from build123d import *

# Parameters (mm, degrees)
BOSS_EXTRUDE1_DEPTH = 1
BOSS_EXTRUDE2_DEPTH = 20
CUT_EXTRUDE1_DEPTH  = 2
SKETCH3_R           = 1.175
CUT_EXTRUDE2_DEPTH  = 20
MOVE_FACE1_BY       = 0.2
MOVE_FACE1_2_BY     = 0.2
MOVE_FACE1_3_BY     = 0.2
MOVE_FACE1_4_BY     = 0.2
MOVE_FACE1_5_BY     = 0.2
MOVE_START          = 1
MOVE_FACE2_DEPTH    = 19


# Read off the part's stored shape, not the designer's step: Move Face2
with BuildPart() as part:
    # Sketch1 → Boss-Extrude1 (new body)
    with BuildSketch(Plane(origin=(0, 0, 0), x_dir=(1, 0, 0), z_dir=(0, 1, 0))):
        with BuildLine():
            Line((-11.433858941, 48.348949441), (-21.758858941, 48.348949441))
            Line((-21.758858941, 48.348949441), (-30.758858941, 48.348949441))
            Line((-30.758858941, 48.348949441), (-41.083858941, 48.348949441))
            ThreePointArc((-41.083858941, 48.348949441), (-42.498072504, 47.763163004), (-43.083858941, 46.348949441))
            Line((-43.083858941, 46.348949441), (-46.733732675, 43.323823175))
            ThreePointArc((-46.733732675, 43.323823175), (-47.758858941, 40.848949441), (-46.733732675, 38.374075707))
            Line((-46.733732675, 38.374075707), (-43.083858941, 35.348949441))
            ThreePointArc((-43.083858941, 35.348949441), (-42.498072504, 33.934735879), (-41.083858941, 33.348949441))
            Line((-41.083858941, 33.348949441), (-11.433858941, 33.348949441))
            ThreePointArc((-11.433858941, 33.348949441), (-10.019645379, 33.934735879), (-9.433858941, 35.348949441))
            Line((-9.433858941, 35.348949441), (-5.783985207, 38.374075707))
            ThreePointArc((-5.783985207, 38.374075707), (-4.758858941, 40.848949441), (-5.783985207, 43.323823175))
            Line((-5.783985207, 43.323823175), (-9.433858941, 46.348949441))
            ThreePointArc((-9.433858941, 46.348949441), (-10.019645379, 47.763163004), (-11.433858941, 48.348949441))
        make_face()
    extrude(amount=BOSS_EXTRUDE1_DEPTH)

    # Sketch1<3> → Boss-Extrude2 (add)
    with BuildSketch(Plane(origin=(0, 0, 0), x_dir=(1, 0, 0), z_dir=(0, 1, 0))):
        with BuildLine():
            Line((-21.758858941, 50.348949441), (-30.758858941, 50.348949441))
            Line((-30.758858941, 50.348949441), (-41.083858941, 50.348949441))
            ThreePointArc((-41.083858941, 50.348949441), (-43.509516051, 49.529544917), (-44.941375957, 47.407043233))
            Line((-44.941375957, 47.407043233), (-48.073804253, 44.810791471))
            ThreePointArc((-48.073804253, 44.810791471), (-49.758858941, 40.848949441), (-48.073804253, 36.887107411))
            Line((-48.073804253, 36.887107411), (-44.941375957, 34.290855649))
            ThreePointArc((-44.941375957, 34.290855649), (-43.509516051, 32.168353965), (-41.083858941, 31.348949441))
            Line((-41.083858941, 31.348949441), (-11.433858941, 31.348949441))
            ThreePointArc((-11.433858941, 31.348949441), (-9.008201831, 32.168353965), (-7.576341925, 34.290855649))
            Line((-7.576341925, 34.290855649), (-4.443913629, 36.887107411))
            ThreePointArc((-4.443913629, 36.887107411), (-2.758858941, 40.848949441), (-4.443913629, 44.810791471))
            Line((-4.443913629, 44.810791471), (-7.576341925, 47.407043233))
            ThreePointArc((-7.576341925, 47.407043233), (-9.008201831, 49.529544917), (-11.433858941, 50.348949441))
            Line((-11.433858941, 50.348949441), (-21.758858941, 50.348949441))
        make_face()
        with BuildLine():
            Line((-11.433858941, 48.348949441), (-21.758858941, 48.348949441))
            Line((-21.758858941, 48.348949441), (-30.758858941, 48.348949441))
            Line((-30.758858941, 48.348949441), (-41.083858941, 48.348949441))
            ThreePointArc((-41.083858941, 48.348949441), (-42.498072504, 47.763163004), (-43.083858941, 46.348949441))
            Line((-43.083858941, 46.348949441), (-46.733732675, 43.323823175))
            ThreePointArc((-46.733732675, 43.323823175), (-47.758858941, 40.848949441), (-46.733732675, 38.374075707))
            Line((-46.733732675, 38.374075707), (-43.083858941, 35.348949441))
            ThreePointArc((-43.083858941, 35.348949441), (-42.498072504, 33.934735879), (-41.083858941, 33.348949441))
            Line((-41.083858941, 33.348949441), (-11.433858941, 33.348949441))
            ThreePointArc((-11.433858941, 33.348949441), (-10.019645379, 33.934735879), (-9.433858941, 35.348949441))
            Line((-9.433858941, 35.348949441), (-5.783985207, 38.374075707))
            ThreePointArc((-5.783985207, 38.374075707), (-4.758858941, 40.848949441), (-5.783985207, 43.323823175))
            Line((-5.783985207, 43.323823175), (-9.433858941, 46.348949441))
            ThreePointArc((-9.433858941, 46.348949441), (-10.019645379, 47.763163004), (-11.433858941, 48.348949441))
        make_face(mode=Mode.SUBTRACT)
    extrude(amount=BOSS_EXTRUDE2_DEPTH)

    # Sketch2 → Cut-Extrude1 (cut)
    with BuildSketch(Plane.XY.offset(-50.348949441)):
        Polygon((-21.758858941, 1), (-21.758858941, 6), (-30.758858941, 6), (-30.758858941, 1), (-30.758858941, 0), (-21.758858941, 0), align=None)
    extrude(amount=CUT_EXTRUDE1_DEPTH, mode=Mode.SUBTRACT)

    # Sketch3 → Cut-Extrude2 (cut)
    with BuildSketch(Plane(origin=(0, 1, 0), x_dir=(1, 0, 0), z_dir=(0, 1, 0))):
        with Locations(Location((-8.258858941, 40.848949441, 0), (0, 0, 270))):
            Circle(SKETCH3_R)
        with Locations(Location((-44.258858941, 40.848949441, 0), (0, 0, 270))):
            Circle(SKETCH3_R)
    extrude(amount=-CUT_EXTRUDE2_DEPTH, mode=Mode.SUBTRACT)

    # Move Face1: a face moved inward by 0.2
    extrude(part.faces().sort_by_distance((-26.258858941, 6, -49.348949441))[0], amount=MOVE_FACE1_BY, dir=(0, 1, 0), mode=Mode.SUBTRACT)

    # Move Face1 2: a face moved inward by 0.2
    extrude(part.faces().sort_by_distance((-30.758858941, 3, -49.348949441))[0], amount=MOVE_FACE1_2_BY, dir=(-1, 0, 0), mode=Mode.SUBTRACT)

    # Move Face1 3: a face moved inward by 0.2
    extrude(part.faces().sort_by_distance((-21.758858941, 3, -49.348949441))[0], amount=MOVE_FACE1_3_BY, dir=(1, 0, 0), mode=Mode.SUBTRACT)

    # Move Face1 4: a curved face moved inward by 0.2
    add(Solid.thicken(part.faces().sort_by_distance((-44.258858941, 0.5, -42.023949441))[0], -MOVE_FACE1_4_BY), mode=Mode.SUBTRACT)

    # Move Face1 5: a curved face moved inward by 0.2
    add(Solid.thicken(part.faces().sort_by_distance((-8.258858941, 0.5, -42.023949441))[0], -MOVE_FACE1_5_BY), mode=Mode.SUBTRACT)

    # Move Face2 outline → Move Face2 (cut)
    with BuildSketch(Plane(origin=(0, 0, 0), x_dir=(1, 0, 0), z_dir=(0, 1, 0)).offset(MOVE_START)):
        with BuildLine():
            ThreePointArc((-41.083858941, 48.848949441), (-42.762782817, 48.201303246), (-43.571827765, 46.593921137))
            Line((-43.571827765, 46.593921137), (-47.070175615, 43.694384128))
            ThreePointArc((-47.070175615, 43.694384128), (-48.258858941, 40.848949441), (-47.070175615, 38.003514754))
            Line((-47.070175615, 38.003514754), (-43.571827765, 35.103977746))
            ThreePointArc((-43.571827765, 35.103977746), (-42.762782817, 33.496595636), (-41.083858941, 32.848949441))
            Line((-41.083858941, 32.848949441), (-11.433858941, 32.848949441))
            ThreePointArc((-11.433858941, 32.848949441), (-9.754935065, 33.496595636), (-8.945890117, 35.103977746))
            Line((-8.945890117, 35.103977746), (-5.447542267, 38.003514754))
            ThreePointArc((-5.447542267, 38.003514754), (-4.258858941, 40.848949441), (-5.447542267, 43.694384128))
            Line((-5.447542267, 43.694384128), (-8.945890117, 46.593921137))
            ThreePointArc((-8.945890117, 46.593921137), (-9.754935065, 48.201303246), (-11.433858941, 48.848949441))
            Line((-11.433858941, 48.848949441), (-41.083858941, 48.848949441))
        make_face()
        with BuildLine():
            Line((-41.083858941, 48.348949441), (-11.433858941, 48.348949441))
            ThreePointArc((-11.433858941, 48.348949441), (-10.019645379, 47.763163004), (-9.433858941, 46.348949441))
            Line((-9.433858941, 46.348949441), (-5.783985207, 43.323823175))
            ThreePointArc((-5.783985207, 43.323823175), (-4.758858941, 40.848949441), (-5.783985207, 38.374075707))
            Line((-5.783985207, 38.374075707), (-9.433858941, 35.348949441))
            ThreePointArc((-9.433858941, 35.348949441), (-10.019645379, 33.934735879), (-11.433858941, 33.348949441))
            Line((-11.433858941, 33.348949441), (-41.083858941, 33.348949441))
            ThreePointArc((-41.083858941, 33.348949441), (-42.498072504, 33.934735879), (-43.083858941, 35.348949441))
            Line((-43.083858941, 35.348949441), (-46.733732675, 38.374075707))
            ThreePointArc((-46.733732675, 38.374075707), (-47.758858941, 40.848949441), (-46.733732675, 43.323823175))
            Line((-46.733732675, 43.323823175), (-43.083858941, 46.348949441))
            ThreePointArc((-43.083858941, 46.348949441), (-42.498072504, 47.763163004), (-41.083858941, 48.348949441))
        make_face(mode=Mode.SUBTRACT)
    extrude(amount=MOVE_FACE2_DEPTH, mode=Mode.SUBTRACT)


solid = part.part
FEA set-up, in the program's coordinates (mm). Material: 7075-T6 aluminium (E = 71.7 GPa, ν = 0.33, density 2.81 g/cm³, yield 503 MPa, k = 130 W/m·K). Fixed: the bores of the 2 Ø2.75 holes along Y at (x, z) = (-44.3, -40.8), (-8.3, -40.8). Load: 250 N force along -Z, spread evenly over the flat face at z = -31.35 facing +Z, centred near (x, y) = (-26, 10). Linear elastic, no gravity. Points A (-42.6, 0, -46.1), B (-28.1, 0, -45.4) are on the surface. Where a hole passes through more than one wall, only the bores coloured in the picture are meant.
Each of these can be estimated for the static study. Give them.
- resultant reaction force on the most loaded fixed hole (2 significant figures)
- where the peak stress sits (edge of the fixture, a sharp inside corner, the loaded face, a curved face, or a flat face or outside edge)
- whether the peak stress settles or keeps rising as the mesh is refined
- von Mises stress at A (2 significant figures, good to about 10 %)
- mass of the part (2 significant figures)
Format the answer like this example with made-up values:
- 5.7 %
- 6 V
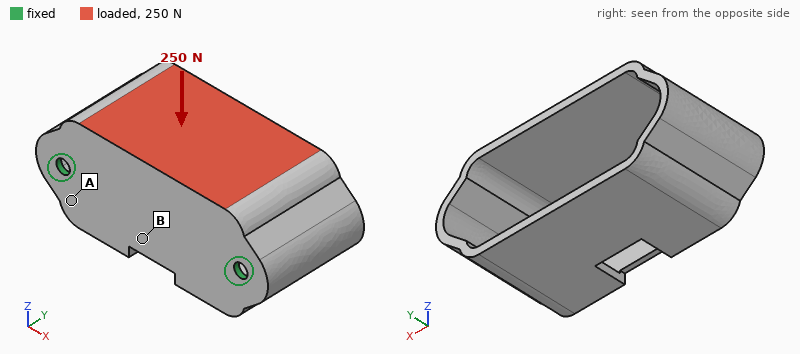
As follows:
- 130 N
- edge of the fixture
- keeps rising
- 59 MPa
- 11 g
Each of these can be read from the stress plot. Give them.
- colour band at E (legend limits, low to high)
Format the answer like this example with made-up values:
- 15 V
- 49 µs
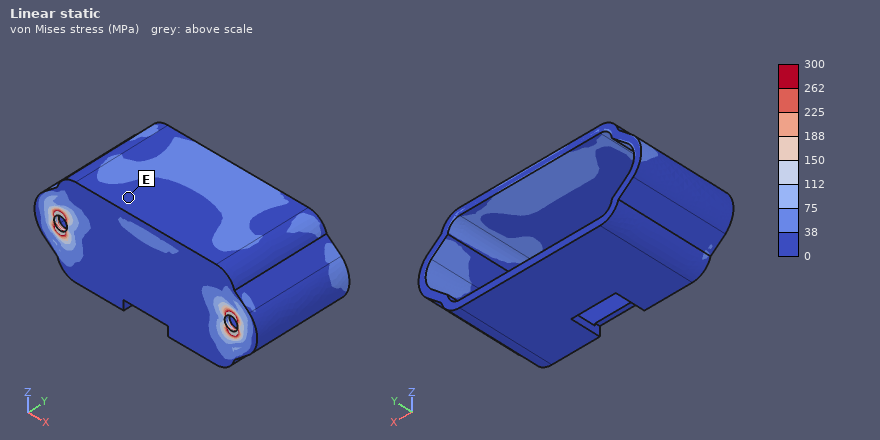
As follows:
- 0 to 38 MPa
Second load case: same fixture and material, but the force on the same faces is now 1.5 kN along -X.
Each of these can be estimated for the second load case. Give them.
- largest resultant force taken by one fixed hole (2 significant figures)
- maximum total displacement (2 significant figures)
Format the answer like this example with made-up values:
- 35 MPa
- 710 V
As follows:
- 910 N
- 0.21 mm
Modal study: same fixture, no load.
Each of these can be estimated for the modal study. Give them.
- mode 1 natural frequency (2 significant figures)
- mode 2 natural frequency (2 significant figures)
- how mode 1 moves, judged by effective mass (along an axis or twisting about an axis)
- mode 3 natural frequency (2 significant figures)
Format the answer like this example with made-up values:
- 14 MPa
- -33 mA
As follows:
- 1900 Hz
- 3900 Hz
- along Z
- 4400 Hz
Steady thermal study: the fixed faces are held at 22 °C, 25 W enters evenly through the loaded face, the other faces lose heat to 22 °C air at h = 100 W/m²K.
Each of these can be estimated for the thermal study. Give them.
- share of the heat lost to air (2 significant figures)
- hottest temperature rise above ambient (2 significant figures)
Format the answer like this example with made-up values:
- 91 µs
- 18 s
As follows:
- 40 %
- 49 K
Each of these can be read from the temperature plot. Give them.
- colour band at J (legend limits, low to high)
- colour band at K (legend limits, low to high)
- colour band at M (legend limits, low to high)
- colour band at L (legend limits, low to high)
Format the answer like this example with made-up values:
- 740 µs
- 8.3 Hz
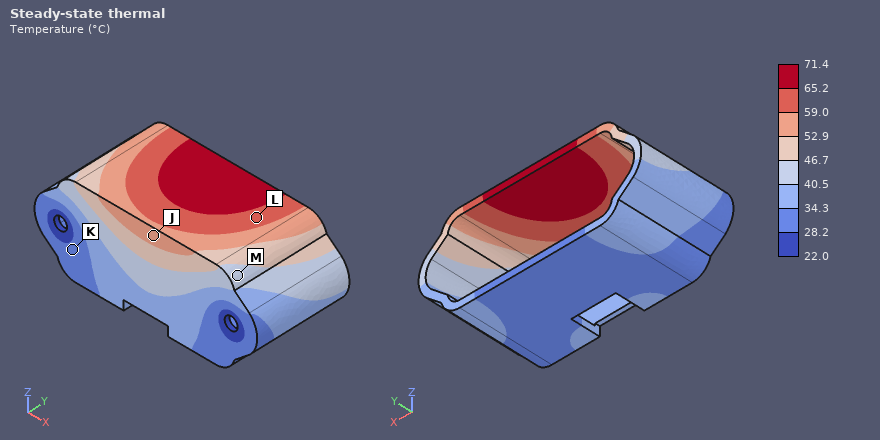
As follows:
- 52.9 to 59.0 °C
- 28.2 to 34.3 °C
- 40.5 to 46.7 °C
- 59.0 to 65.2 °C
